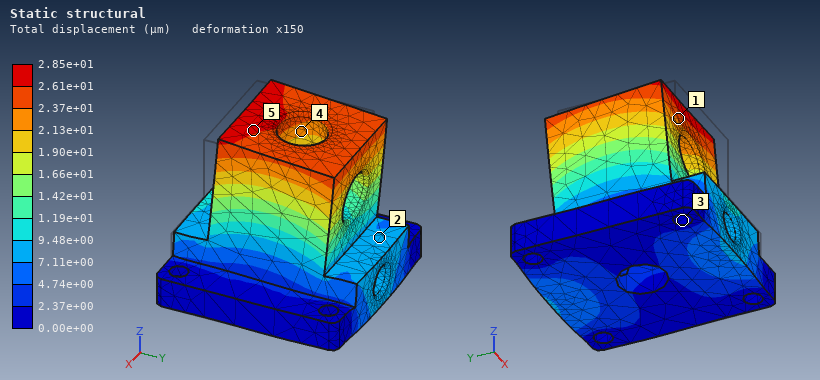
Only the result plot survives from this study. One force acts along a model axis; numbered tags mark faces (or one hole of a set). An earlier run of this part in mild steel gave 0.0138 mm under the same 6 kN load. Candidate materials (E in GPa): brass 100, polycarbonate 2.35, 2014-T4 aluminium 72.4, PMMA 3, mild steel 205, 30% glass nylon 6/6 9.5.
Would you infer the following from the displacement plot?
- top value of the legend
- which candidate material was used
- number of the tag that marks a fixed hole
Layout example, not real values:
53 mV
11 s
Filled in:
2.85e+01 µm
brass
3
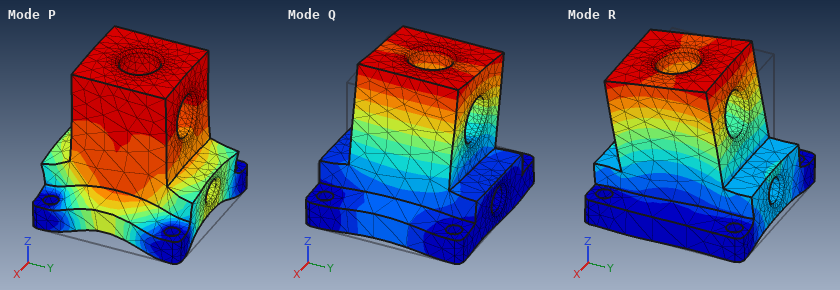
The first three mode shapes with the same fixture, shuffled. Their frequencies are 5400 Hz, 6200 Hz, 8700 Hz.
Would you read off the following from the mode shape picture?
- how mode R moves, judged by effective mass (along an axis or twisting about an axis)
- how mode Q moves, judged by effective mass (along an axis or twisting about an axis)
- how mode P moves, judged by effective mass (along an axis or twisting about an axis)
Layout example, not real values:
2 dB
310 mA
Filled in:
along Y
along X
along Z
